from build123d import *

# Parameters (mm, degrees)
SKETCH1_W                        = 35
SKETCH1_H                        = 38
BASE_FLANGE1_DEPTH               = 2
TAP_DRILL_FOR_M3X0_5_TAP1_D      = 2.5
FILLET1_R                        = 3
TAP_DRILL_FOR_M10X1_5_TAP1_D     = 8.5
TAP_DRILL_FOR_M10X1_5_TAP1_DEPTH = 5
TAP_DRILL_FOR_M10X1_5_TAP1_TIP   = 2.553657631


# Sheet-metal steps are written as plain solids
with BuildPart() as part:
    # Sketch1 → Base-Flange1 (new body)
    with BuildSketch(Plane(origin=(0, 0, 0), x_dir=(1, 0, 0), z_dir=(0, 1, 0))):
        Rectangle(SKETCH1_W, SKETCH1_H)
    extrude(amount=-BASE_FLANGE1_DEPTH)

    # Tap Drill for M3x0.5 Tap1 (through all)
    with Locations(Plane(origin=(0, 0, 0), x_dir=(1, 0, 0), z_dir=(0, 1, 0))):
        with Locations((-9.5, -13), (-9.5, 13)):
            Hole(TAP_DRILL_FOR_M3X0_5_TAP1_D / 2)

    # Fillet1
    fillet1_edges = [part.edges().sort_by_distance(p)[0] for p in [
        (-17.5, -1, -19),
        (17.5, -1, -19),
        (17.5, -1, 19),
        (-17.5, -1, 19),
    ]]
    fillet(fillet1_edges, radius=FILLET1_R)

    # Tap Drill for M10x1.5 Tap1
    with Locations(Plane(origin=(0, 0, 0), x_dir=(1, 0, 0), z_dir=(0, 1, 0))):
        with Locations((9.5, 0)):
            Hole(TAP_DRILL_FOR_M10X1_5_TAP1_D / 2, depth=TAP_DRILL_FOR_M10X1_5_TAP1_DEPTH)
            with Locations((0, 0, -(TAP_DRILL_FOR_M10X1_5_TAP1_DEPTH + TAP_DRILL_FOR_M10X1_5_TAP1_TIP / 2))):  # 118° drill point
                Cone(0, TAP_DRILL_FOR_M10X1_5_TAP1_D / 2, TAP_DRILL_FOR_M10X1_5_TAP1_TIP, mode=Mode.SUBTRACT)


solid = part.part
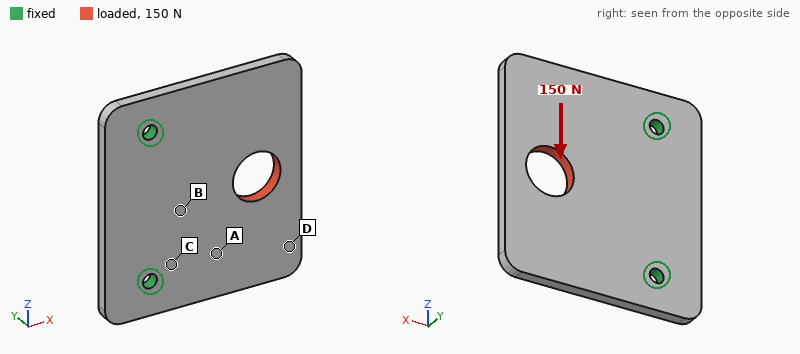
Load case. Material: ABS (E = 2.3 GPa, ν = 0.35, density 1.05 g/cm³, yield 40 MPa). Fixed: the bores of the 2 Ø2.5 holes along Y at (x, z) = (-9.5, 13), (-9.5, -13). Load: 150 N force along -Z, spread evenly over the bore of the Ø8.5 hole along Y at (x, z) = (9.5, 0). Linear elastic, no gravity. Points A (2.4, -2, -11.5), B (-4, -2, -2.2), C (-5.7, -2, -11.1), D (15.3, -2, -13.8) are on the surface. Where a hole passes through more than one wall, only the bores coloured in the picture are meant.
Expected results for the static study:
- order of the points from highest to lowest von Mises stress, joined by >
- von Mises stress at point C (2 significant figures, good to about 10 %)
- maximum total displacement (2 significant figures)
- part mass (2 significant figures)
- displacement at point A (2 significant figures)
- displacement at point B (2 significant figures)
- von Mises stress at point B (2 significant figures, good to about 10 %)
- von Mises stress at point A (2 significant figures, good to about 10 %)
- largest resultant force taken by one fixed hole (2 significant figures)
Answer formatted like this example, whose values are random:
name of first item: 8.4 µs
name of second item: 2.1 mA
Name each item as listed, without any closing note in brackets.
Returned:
order of the points from highest to lowest von Mises stress, joined by >: C > B > A > D
von Mises stress at point C: 6.5 MPa
maximum total displacement: 0.12 mm
part mass: 2.6 g
displacement at point A: 0.053 mm
displacement at point B: 0.025 mm
von Mises stress at point B: 4.8 MPa
von Mises stress at point A: 3.3 MPa
largest resultant force taken by one fixed hole: 130 N
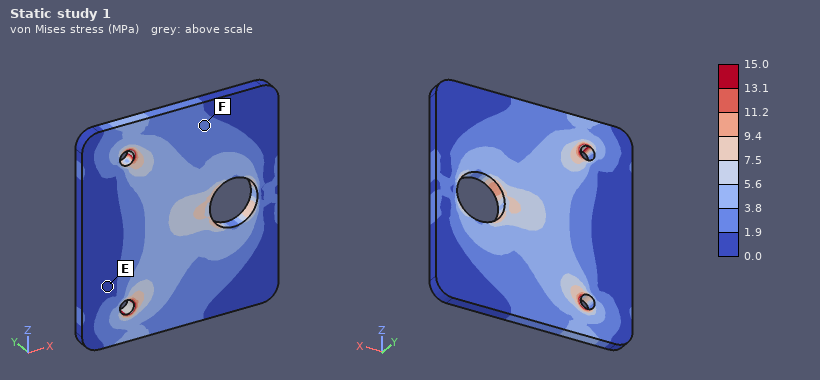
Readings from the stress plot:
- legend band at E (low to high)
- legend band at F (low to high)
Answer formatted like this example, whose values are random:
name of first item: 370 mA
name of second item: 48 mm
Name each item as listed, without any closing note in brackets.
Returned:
legend band at E: 0.0 to 1.9 MPa
legend band at F: 1.9 to 3.8 MPa
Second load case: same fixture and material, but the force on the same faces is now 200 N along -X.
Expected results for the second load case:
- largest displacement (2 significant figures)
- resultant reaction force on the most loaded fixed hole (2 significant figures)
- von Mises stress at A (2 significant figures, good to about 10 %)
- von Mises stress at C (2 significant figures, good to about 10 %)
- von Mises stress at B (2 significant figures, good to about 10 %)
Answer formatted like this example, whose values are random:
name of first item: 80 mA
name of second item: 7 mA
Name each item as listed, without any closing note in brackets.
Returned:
largest displacement: 74 µm
resultant reaction force on the most loaded fixed hole: 100 N
von Mises stress at A: 3.4 MPa
von Mises stress at C: 6.0 MPa
von Mises stress at B: 2.2 MPa
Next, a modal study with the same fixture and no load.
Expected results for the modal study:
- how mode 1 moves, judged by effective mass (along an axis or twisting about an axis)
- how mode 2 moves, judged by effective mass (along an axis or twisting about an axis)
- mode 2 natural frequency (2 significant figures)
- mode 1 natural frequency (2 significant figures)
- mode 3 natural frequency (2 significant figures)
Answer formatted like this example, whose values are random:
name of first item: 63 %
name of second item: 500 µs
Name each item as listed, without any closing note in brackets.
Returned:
how mode 1 moves, judged by effective mass: along Y
how mode 2 moves, judged by effective mass: twisting about X
mode 2 natural frequency: 1200 Hz
mode 1 natural frequency: 640 Hz
mode 3 natural frequency: 2700 Hz
